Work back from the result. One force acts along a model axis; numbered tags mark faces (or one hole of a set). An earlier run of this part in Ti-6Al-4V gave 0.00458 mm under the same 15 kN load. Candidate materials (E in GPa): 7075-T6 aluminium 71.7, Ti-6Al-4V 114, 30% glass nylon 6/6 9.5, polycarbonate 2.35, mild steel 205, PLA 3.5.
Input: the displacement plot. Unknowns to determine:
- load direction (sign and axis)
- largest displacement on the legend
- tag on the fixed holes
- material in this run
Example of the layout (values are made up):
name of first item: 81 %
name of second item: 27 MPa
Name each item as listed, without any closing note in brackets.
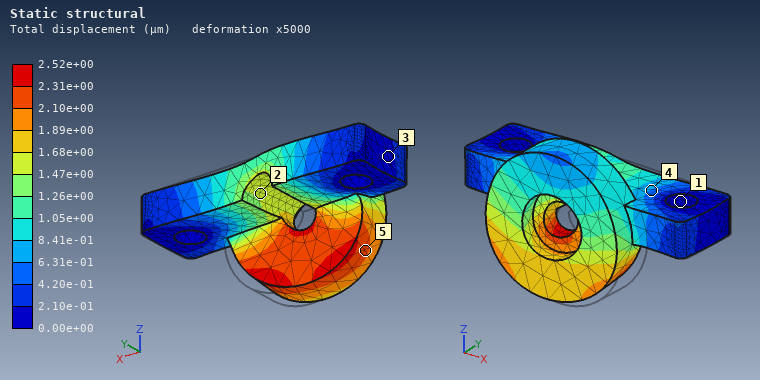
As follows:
load direction: -X
largest displacement on the legend: 2.52e+00 µm
tag on the fixed holes: 1
material in this run: mild steel
